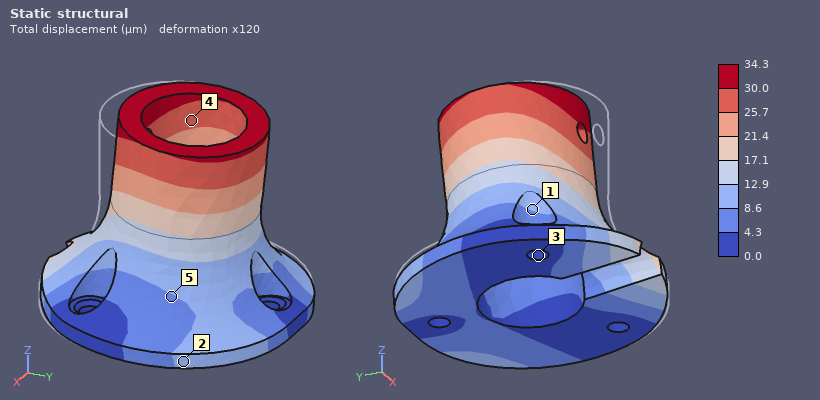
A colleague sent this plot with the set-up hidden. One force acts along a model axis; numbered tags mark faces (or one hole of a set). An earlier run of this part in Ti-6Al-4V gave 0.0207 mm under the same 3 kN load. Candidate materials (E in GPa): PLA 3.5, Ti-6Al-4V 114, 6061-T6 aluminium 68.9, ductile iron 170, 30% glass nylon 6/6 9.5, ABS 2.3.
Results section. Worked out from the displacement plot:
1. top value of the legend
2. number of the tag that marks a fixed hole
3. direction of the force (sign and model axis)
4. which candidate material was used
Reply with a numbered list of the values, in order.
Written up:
1. 34.3 µm
2. 3
3. +Y
4. 6061-T6 aluminium
